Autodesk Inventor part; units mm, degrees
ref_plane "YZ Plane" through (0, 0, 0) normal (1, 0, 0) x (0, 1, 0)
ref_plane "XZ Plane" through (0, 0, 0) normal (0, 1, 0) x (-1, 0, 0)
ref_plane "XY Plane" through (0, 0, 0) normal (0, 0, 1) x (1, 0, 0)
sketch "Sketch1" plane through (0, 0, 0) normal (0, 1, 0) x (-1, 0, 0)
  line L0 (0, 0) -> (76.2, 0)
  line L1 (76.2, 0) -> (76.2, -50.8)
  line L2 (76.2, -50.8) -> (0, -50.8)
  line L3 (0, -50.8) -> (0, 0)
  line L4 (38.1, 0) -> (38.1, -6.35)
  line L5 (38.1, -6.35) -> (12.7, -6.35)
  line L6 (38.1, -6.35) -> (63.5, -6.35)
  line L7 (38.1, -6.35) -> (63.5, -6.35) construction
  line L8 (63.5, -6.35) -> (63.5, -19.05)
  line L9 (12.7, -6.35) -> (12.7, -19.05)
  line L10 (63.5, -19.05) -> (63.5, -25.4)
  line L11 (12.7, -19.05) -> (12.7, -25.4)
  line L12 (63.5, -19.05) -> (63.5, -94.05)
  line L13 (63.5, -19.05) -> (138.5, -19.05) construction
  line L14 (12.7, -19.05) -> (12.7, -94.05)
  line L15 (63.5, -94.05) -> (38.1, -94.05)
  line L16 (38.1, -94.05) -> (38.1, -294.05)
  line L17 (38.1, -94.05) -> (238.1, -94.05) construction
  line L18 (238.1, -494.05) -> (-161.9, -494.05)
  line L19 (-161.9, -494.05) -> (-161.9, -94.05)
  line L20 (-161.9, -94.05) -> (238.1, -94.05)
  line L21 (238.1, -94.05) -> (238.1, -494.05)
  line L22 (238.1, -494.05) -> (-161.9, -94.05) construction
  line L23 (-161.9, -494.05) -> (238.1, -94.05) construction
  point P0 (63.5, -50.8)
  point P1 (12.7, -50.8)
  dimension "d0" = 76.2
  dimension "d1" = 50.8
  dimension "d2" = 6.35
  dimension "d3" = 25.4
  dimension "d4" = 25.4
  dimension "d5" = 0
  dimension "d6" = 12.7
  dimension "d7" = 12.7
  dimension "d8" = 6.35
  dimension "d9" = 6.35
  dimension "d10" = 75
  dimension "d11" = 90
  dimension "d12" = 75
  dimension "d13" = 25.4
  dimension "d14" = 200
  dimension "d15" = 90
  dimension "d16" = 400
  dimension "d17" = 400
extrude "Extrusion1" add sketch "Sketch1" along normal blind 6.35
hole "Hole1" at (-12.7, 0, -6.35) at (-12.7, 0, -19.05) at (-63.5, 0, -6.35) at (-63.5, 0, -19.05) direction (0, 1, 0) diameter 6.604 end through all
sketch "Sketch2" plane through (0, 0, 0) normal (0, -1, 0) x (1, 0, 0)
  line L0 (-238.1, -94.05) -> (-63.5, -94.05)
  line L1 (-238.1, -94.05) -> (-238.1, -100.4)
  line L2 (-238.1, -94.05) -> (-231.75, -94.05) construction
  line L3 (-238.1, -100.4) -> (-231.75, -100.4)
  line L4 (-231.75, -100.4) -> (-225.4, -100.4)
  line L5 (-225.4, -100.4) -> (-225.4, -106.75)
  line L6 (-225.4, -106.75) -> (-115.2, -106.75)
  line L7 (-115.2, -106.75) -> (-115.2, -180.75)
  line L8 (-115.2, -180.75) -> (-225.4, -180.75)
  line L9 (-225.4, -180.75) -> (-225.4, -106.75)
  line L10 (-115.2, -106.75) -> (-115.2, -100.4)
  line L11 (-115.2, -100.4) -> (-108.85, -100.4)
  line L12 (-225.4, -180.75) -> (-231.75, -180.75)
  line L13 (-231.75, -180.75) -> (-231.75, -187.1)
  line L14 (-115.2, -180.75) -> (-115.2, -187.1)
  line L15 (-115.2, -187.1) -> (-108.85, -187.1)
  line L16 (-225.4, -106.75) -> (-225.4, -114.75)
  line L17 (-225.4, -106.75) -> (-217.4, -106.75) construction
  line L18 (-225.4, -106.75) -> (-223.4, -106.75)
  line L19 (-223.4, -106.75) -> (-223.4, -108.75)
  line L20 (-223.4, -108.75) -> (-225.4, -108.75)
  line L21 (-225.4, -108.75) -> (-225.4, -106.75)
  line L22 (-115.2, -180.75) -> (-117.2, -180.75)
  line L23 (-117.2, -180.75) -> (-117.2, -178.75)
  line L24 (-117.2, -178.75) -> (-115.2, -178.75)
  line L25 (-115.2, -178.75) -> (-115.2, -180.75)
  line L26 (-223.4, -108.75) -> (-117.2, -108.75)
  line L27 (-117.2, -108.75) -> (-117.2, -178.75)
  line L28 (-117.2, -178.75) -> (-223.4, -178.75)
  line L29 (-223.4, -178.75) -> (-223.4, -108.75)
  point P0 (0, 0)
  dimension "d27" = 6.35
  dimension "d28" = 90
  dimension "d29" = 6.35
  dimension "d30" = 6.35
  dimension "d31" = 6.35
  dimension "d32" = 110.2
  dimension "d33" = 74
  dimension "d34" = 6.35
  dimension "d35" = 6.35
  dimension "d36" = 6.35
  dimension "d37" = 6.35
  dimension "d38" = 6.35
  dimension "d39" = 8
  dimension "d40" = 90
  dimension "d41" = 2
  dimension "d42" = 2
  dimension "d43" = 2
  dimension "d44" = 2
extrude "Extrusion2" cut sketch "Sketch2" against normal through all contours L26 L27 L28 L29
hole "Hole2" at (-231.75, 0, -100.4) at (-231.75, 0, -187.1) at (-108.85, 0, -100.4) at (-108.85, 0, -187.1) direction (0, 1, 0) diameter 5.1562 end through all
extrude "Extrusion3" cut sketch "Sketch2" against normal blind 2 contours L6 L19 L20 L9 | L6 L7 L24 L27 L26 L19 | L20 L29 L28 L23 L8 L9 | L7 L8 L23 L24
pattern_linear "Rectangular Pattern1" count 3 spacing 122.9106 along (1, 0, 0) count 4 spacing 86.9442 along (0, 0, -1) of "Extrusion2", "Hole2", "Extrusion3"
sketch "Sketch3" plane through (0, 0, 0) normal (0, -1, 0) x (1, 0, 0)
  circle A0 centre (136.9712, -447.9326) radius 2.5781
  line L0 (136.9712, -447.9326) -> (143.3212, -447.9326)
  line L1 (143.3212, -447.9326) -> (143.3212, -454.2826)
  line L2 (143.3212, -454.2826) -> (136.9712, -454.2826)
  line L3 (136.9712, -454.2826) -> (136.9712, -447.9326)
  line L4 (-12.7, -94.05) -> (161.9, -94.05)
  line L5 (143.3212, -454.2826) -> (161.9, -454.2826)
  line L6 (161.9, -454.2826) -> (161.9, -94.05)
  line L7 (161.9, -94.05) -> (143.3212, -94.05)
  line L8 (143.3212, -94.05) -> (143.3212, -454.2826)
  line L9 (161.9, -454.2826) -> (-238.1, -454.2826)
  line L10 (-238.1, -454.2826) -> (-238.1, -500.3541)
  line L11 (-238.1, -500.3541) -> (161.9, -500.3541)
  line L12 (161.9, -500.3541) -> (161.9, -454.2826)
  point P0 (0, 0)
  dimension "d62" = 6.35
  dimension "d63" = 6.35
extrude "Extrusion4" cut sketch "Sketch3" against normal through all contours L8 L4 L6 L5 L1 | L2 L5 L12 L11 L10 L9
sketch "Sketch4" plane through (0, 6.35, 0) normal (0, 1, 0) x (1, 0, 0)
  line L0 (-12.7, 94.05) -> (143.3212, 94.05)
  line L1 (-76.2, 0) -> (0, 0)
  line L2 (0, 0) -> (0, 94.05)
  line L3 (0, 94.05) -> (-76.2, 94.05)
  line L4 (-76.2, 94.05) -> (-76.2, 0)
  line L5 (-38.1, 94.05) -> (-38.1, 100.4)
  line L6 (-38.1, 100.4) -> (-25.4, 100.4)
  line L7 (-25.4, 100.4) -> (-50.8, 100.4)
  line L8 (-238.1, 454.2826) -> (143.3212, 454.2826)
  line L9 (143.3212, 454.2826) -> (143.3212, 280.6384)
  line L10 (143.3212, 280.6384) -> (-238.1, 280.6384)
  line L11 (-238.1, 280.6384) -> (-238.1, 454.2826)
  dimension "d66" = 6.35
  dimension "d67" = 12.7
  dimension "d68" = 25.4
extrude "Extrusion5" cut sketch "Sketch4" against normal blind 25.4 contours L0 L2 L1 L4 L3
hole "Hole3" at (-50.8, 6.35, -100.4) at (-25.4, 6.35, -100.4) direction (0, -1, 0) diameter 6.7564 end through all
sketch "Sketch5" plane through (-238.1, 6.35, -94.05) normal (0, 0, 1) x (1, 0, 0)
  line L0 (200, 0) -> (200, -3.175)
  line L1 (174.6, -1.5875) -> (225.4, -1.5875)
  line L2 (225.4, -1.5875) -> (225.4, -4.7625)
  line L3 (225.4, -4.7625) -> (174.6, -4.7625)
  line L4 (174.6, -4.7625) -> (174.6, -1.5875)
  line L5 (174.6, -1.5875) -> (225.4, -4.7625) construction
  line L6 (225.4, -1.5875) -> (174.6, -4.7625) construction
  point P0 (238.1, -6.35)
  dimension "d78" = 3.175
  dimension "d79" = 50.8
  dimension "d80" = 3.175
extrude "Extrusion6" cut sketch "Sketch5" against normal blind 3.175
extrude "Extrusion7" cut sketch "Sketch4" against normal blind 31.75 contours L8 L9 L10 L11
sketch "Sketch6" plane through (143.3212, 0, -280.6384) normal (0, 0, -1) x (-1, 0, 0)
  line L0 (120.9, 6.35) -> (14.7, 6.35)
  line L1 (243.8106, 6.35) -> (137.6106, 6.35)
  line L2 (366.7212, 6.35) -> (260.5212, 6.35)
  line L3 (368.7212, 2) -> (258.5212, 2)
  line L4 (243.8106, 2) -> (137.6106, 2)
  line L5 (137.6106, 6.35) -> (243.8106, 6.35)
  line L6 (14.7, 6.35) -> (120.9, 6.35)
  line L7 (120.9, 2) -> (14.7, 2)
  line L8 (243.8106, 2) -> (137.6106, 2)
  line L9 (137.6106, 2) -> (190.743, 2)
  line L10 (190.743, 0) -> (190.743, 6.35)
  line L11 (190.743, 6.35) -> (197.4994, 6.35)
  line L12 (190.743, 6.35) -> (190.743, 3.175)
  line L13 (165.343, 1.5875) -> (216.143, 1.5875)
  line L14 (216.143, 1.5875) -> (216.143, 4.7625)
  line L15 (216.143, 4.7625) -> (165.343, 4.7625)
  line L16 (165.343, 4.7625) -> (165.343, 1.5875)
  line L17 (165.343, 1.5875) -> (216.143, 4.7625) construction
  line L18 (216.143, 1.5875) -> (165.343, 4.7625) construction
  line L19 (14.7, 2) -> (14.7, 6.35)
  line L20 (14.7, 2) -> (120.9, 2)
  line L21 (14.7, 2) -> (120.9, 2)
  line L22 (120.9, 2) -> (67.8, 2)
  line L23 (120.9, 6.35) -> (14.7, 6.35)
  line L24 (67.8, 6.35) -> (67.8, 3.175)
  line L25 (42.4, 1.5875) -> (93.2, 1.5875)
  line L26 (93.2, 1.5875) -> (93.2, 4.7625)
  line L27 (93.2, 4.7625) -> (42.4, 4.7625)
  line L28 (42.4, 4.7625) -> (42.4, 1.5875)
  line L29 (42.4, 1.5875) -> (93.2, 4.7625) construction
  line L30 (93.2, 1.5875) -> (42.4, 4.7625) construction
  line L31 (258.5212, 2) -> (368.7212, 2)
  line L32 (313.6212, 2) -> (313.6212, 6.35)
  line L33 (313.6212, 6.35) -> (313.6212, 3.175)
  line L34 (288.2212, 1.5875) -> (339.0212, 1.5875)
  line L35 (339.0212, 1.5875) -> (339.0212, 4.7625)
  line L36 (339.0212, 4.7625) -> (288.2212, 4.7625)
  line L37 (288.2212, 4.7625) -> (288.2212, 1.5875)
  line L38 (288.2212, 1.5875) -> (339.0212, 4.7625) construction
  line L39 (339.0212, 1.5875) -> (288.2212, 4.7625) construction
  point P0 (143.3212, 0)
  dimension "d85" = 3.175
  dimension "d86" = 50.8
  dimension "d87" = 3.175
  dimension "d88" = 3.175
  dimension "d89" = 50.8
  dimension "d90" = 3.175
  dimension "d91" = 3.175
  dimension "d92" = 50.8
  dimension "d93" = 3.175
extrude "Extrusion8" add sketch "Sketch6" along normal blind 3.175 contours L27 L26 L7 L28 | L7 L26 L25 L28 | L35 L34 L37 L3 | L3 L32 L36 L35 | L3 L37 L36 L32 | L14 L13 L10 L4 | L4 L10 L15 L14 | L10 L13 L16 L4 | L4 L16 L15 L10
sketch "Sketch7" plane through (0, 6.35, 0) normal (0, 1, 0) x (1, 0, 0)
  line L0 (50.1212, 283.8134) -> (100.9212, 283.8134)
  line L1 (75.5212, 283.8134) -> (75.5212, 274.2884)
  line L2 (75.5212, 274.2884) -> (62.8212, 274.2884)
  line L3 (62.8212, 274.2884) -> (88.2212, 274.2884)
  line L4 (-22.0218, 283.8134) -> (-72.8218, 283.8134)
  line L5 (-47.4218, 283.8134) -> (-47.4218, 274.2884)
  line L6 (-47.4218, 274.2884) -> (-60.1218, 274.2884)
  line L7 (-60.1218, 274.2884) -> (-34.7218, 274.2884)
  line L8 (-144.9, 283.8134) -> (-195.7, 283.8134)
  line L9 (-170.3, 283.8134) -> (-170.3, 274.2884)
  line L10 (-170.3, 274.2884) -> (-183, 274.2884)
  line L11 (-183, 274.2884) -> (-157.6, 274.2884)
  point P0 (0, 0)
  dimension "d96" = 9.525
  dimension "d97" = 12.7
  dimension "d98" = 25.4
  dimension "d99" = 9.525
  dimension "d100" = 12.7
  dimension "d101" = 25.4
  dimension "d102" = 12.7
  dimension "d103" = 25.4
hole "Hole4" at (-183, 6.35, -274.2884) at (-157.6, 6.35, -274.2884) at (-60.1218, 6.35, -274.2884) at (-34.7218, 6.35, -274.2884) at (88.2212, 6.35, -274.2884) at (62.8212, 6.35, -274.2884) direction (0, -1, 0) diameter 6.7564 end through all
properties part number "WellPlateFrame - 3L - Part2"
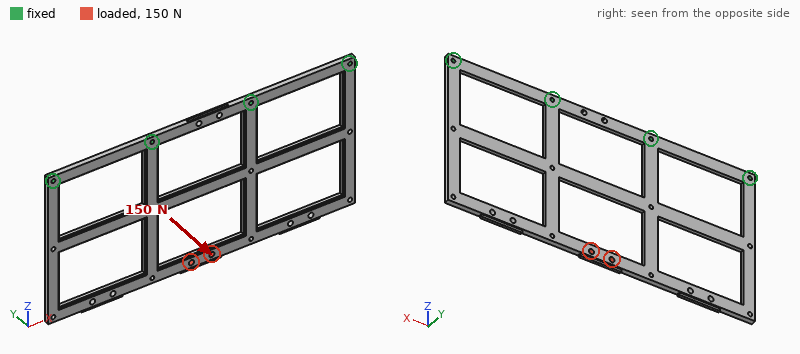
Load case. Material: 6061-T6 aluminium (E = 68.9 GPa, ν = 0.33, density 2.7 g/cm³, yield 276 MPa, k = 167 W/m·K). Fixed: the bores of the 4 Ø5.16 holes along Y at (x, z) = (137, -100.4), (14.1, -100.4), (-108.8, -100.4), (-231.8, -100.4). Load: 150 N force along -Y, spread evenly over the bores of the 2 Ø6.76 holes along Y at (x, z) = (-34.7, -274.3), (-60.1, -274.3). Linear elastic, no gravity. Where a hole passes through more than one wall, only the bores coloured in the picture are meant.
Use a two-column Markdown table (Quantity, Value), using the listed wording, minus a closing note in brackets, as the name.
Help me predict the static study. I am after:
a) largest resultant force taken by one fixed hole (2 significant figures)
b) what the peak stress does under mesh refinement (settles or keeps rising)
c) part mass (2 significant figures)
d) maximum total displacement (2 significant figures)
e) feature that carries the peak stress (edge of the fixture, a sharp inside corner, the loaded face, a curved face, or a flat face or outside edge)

| Quantity | Value |
|---|---|
| largest resultant force taken by one fixed hole | 64 N |
| what the peak stress does under mesh refinement | keeps rising |
| part mass | 430 g |
| maximum total displacement | 4.0 mm |
| feature that carries the peak stress | edge of the fixture |
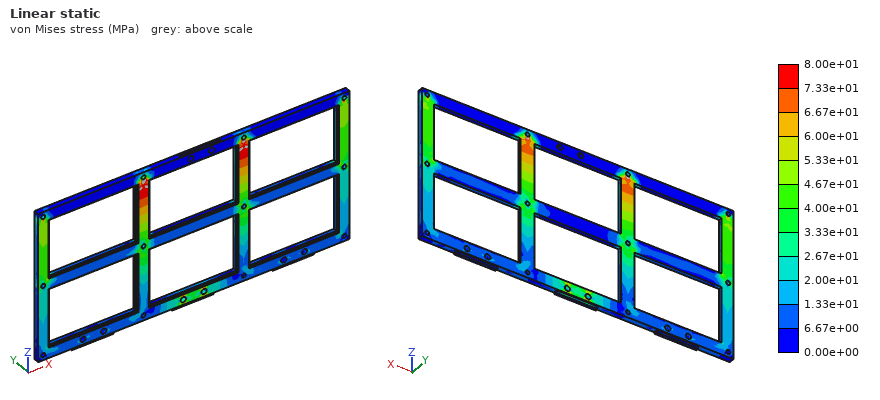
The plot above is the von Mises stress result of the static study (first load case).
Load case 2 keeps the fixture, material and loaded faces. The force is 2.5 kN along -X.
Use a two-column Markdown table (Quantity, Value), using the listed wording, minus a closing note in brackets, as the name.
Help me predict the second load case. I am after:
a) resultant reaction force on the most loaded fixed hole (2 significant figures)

| Quantity | Value |
|---|---|
| resultant reaction force on the most loaded fixed hole | 1.1 kN |
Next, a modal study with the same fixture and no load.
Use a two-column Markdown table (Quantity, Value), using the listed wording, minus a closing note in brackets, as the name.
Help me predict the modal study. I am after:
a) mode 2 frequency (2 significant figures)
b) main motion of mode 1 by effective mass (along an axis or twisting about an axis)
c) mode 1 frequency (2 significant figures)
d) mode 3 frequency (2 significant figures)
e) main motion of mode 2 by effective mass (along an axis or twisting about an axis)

| Quantity | Value |
|---|---|
| mode 2 frequency | 170 Hz |
| main motion of mode 1 by effective mass | along Y |
| mode 1 frequency | 96 Hz |
| mode 3 frequency | 310 Hz |
| main motion of mode 2 by effective mass | twisting about Z |
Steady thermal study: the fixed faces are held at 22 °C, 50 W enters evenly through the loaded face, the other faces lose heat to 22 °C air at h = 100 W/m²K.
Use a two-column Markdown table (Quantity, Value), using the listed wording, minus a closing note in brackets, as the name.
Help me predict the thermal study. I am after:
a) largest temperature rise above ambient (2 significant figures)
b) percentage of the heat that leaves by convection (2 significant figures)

| Quantity | Value |
|---|---|
| largest temperature rise above ambient | 73 K |
| percentage of the heat that leaves by convection | 98 % |
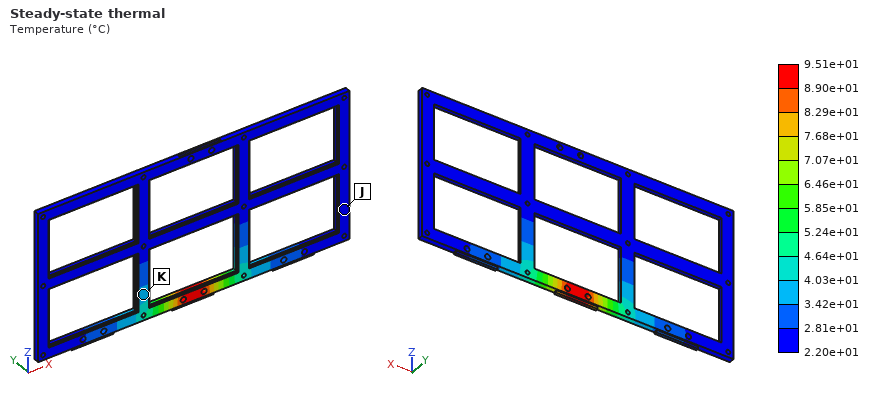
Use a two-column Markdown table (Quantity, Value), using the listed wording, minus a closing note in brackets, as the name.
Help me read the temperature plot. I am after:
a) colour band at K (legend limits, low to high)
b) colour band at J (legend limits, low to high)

| Quantity | Value |
|---|---|
| colour band at K | 3.42e+01 to 4.03e+01 °C |
| colour band at J | 2.20e+01 to 2.81e+01 °C |
